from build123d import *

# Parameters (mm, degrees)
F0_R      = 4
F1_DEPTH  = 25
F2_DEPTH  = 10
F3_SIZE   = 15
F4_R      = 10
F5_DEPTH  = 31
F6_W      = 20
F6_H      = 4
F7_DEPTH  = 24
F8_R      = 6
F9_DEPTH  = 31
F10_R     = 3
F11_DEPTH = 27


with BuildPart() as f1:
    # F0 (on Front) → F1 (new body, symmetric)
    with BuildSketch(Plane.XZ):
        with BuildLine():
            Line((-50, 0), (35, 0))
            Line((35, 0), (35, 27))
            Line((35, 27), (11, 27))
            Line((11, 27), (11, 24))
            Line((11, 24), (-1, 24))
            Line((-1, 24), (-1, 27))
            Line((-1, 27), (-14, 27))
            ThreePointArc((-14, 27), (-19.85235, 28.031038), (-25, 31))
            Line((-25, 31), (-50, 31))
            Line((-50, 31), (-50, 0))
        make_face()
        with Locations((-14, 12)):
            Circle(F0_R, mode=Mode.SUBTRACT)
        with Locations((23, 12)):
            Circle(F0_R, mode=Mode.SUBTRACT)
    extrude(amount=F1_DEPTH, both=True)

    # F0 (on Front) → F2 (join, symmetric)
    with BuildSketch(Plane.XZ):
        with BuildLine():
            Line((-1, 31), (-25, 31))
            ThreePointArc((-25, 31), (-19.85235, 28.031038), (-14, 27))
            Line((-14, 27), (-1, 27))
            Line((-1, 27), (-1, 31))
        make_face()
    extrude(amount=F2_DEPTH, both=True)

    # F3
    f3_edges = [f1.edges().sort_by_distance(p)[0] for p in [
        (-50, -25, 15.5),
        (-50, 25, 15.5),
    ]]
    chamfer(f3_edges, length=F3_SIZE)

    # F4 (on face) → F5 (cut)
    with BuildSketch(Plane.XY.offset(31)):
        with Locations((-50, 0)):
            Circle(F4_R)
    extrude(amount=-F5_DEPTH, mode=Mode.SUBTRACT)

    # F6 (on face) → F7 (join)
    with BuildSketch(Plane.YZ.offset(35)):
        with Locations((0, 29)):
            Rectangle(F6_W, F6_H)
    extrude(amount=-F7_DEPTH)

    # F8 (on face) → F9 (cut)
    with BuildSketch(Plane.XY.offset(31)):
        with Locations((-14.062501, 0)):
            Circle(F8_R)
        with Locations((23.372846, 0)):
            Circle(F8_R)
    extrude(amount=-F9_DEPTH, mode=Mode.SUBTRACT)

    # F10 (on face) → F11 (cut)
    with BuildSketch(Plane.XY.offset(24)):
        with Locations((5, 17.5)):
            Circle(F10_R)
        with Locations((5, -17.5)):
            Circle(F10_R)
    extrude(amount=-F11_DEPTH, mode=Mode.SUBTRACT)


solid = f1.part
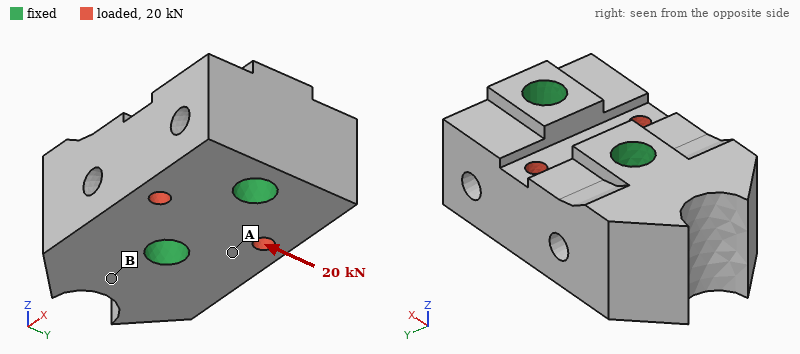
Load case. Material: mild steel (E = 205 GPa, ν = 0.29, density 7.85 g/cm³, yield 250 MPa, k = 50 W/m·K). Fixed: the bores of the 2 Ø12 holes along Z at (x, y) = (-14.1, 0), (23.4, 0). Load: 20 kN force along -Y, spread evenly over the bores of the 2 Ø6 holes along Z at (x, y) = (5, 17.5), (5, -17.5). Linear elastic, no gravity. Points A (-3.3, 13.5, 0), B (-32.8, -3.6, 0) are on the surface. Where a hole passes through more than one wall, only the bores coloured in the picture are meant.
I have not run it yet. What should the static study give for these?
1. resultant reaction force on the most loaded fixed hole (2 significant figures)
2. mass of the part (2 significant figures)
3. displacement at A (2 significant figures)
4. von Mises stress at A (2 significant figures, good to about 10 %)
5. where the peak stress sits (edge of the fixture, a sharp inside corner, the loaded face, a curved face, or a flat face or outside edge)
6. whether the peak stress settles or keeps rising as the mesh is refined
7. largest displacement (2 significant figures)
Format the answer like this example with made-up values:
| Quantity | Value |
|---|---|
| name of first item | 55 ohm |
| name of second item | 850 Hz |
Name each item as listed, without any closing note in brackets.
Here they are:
| Quantity | Value |
|---|---|
| resultant reaction force on the most loaded fixed hole | 10 kN |
| mass of the part | 770 g |
| displacement at A | 1.4 µm |
| von Mises stress at A | 19 MPa |
| where the peak stress sits | edge of the fixture |
| whether the peak stress settles or keeps rising as the mesh is refined | keeps rising |
| largest displacement | 3.2 µm |
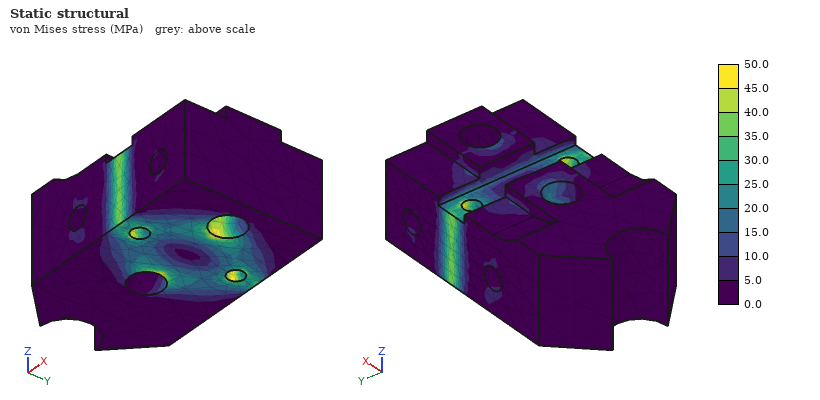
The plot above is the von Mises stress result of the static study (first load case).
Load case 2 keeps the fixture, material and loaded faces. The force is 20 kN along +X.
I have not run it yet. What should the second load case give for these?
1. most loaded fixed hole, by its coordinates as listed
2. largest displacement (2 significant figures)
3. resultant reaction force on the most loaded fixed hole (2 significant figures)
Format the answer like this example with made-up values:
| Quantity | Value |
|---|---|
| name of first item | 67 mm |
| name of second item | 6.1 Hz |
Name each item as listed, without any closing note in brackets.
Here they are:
| Quantity | Value |
|---|---|
| most loaded fixed hole, by its coordinates as listed | (-14.1, 0) |
| largest displacement | 2.4 µm |
| resultant reaction force on the most loaded fixed hole | 11 kN |
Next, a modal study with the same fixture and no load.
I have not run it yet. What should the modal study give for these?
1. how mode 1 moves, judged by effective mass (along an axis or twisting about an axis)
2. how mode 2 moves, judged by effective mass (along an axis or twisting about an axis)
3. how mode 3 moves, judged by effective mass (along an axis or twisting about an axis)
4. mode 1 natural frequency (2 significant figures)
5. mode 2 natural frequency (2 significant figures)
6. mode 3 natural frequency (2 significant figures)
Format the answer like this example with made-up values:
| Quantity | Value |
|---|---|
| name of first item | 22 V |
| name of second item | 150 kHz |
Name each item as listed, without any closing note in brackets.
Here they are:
| Quantity | Value |
|---|---|
| how mode 1 moves, judged by effective mass | along Y |
| how mode 2 moves, judged by effective mass | along Z |
| how mode 3 moves, judged by effective mass | twisting about X |
| mode 1 natural frequency | 15 kHz |
| mode 2 natural frequency | 17 kHz |
| mode 3 natural frequency | 19 kHz |
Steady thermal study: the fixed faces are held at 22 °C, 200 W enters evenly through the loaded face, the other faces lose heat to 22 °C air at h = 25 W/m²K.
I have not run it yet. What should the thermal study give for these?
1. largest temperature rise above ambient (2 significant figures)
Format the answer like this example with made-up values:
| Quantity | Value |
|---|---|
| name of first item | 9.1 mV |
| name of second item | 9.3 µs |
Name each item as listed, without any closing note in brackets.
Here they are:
| Quantity | Value |
|---|---|
| largest temperature rise above ambient | 50 K |
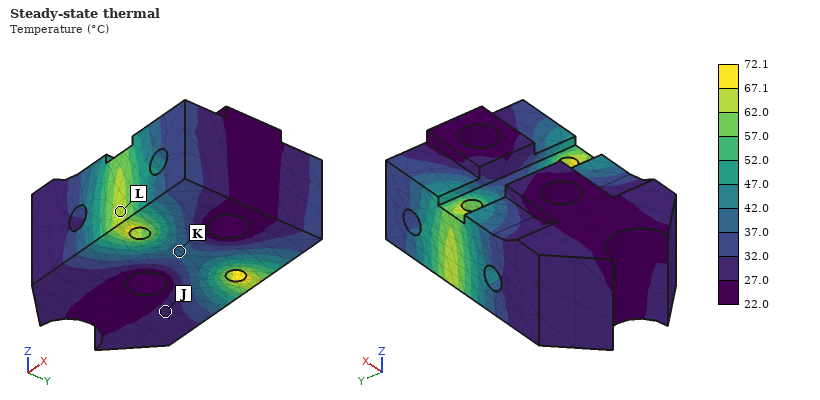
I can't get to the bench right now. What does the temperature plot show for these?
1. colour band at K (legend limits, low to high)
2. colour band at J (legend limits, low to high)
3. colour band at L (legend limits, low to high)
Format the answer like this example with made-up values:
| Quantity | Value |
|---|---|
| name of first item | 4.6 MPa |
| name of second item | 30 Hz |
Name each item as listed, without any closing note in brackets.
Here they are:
| Quantity | Value |
|---|---|
| colour band at K | 37.0 to 42.0 °C |
| colour band at J | 27.0 to 32.0 °C |
| colour band at L | 62.0 to 67.1 °C |
